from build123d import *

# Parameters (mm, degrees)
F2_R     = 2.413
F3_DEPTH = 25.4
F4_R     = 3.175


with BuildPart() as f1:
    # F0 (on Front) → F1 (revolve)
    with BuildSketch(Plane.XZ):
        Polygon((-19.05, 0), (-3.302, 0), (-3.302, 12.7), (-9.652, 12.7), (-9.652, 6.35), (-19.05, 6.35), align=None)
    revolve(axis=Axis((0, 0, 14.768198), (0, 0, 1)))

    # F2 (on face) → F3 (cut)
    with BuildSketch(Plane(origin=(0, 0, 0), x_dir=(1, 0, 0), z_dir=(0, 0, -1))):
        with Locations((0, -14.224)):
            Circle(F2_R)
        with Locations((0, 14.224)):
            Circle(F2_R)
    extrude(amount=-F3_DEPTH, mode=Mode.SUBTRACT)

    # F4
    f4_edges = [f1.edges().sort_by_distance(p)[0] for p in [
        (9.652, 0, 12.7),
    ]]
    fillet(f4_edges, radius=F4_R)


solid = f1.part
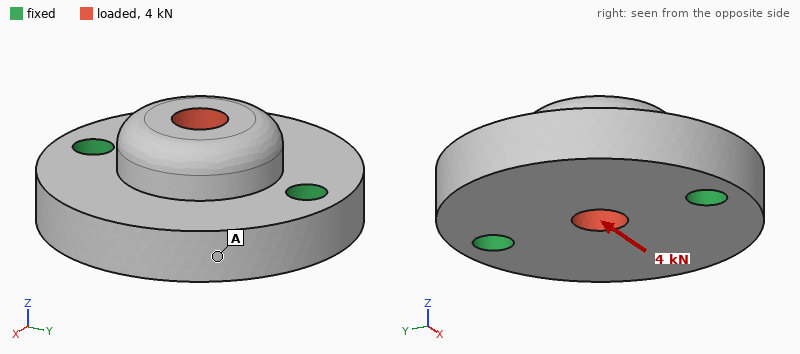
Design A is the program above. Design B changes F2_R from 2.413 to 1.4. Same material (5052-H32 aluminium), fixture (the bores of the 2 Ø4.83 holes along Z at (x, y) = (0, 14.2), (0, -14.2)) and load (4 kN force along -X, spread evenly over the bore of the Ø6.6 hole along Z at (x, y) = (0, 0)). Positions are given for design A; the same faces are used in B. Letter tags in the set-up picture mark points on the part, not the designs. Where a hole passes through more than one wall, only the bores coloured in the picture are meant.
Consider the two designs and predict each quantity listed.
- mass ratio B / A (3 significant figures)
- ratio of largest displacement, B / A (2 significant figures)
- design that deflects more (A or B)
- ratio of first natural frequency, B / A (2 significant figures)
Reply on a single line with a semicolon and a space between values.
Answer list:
1.02; 1.5; B; 0.81
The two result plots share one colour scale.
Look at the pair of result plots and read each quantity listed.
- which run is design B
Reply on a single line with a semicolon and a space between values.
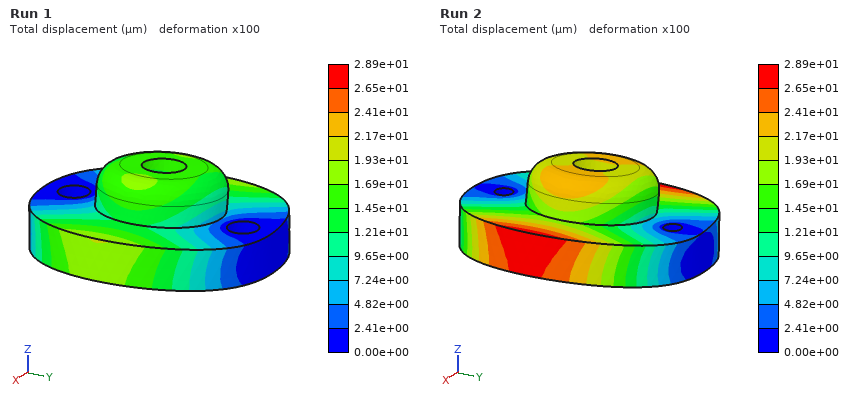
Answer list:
Run 2
